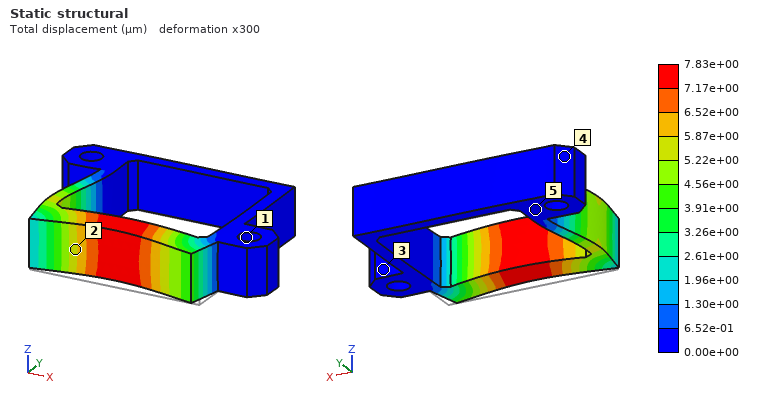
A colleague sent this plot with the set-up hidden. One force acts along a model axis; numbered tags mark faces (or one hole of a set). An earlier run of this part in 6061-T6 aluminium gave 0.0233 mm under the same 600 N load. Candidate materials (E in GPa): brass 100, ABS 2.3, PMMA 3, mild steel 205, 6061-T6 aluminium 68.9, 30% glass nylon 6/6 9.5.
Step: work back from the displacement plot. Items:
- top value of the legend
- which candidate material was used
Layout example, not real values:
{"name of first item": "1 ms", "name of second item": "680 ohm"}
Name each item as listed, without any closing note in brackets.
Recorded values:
{"top value of the legend": "7.83e+00 µm", "which candidate material was used": "mild steel"}
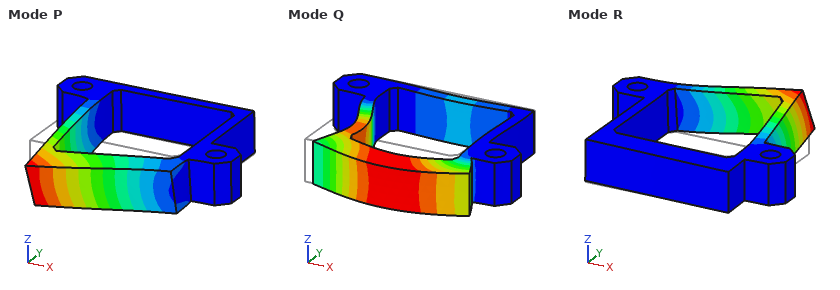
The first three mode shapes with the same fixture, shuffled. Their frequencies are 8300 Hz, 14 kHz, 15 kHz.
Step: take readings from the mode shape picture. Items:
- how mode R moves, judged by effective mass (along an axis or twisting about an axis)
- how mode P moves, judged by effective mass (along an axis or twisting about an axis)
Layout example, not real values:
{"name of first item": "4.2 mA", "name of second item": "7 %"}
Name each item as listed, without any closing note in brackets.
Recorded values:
{"how mode R moves, judged by effective mass": "along Z", "how mode P moves, judged by effective mass": "along Z"}
